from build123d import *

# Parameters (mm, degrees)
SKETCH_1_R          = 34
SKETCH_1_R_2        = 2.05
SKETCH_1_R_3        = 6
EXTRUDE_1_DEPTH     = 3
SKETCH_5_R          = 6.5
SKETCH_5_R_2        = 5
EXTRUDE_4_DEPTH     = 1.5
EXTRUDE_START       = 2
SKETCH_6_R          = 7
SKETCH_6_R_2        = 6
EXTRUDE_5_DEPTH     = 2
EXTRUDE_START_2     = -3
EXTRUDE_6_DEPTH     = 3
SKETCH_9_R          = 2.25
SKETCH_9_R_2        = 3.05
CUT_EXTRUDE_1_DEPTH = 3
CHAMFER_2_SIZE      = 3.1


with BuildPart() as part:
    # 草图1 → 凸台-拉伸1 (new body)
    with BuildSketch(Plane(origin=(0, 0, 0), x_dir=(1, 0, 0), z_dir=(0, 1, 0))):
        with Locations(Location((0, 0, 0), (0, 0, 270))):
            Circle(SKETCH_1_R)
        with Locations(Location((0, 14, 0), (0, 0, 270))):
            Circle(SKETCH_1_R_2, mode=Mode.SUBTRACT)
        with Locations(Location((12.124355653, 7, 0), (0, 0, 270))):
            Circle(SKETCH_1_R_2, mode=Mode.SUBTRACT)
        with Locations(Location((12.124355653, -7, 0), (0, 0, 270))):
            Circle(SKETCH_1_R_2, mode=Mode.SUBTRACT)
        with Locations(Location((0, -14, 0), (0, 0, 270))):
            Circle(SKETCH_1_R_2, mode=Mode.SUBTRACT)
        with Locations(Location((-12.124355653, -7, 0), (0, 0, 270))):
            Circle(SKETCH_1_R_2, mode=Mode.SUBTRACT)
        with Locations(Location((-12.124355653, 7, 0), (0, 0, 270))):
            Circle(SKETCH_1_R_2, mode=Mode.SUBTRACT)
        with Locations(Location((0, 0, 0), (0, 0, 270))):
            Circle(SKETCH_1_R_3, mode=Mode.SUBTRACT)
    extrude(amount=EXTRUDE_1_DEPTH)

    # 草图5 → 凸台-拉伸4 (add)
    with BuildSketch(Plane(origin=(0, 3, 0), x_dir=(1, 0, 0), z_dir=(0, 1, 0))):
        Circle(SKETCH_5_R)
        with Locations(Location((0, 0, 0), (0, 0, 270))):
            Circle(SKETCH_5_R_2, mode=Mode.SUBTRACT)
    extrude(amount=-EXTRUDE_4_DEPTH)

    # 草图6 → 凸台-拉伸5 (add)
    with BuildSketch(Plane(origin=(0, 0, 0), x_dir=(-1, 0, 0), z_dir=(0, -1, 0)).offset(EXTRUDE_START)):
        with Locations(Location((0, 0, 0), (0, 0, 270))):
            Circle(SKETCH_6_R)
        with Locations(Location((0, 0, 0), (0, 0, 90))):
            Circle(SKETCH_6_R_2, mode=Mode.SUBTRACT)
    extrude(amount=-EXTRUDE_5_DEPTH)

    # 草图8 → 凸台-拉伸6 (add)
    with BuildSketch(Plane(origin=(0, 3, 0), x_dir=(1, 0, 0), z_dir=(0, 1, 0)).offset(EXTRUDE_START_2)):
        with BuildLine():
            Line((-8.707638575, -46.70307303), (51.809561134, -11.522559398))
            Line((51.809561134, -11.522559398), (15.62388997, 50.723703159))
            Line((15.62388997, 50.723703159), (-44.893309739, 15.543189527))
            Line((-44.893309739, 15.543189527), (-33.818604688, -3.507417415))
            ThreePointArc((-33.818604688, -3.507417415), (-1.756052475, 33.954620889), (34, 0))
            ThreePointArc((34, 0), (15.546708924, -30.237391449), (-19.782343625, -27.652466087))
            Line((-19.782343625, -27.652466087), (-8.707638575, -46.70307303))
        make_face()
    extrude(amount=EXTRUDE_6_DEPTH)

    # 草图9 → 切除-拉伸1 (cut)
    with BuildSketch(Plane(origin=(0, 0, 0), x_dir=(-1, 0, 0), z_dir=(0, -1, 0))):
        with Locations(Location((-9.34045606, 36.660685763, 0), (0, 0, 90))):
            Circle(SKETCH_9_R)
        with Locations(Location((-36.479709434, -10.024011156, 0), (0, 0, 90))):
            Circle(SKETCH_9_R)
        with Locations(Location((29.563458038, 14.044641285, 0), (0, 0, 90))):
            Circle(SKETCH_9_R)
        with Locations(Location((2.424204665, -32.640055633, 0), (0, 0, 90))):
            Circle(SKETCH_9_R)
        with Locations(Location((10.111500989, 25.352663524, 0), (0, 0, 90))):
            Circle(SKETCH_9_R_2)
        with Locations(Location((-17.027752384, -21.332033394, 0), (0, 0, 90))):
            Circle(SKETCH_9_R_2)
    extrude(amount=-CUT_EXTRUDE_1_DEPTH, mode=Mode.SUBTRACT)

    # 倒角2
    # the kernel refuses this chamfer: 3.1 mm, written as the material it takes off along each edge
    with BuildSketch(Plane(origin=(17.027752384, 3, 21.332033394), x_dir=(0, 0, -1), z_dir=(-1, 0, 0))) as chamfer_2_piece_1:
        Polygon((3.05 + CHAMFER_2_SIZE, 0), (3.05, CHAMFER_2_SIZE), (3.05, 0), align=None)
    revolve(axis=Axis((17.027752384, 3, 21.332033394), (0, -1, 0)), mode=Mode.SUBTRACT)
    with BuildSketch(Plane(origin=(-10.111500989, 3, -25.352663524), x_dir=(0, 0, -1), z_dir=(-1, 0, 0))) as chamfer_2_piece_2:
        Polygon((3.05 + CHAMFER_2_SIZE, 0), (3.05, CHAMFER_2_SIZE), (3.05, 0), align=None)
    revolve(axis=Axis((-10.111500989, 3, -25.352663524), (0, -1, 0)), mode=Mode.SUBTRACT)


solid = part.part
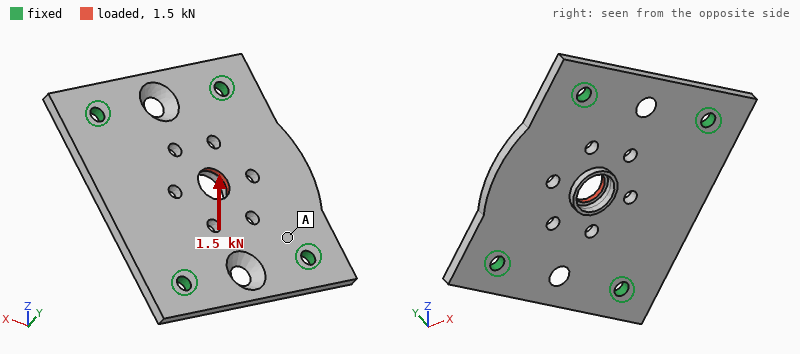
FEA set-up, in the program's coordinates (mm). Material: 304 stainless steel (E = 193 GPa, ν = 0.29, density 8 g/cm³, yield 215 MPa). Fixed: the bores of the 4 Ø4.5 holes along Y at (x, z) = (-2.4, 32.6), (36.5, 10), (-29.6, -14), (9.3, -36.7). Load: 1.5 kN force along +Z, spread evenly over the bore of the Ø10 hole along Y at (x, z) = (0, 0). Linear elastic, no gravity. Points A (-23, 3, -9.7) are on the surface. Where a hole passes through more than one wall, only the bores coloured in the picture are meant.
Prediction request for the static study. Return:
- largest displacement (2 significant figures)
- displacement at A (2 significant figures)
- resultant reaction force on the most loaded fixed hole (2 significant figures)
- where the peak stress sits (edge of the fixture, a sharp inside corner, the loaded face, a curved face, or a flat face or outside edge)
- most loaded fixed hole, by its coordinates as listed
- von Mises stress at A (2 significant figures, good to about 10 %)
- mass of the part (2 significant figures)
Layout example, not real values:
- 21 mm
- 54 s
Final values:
- 2.7 µm
- 0.50 µm
- 550 N
- a sharp inside corner
- (-2.4, 32.6)
- 7.1 MPa
- 110 g
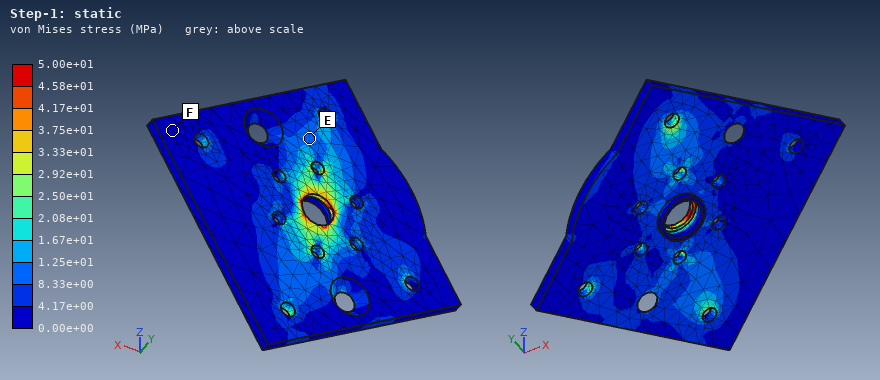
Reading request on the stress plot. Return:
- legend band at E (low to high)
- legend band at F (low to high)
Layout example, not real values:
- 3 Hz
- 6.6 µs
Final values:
- 8.33e+00 to 1.25e+01 MPa
- 0.00e+00 to 4.17e+00 MPa
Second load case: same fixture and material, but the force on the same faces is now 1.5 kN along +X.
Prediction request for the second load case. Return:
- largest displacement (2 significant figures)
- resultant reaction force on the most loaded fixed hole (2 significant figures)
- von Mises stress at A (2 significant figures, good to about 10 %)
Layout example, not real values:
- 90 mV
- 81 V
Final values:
- 2.8 µm
- 530 N
- 13 MPa
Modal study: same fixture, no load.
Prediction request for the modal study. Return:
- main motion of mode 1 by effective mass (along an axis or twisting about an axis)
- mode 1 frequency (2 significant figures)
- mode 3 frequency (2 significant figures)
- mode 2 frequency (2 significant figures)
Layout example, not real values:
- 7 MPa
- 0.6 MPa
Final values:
- along Y
- 4400 Hz
- 6000 Hz
- 5200 Hz
